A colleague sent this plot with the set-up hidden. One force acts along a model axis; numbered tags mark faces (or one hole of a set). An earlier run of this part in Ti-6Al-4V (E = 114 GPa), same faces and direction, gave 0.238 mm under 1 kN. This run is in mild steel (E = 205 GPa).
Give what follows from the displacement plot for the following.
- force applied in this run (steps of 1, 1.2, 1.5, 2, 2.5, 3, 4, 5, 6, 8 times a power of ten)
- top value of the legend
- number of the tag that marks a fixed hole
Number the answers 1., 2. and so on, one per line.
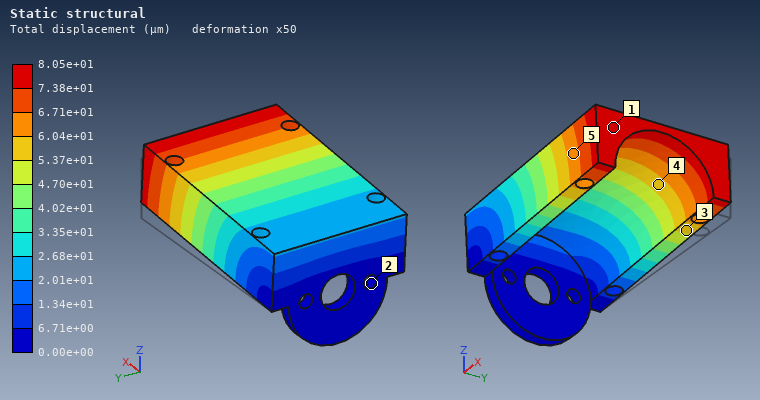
1. 600 N
2. 8.05e+01 µm
3. 2
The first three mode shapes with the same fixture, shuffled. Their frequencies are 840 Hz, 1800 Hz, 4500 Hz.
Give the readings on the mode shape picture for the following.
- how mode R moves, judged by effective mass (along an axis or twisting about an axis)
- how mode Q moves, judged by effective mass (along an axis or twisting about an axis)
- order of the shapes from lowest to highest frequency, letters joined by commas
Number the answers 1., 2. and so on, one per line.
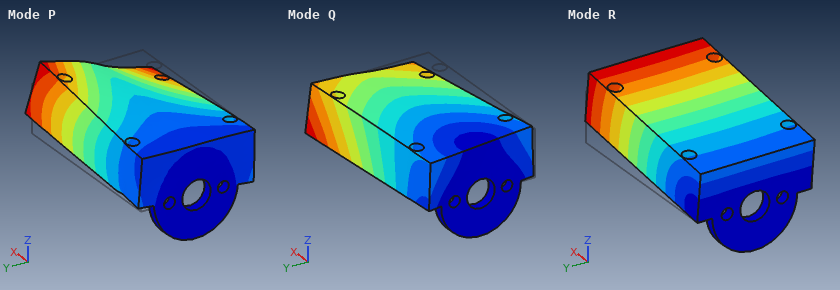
1. along Z
2. along Y
3. R, Q, P
